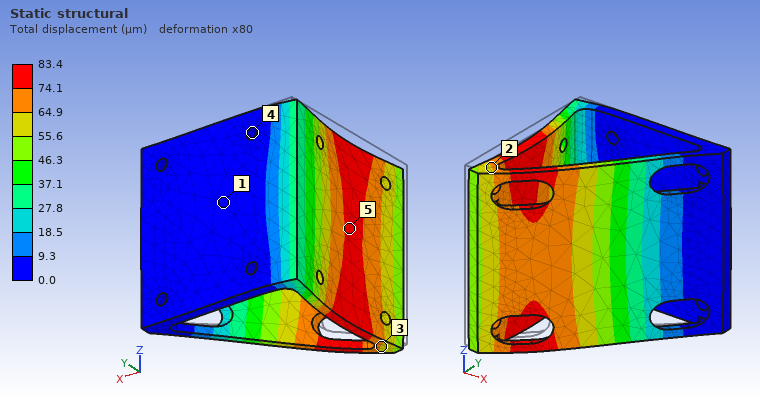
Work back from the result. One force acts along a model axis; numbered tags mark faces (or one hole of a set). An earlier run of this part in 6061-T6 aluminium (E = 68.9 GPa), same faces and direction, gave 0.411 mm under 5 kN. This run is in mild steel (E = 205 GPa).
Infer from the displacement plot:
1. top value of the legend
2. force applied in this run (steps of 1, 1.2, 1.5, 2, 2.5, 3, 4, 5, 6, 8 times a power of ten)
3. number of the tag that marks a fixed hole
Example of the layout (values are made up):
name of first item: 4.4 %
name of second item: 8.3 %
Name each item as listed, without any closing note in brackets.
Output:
top value of the legend: 83.4 µm
force applied in this run: 3 kN
number of the tag that marks a fixed hole: 4
